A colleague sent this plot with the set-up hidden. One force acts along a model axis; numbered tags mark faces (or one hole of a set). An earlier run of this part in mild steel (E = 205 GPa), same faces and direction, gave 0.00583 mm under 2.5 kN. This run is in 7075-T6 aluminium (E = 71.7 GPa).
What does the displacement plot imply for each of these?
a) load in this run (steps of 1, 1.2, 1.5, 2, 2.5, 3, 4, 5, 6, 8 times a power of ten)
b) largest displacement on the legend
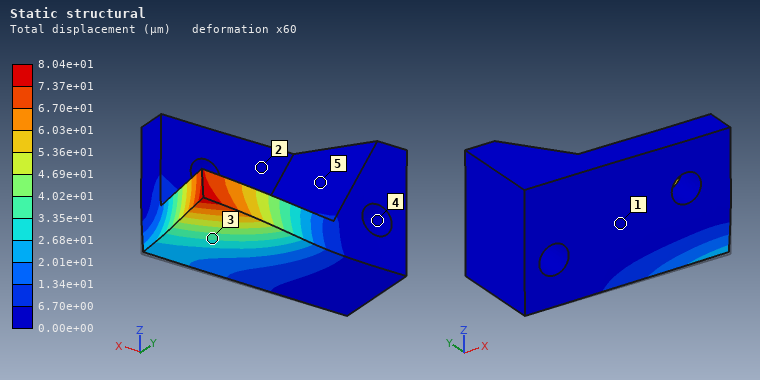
12 kN
8.04e+01 µm
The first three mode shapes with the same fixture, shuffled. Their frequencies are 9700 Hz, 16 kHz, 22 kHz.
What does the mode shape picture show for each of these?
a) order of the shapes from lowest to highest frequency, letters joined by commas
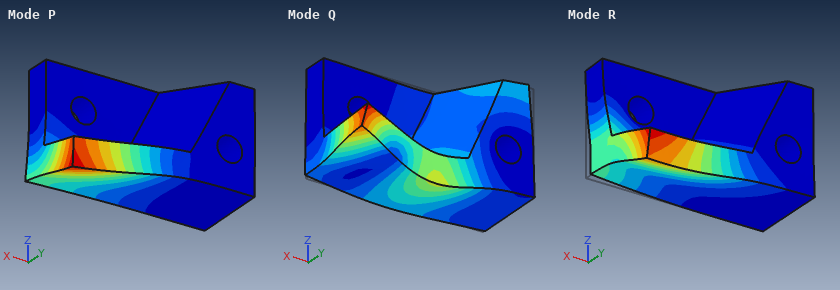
P, R, Q
